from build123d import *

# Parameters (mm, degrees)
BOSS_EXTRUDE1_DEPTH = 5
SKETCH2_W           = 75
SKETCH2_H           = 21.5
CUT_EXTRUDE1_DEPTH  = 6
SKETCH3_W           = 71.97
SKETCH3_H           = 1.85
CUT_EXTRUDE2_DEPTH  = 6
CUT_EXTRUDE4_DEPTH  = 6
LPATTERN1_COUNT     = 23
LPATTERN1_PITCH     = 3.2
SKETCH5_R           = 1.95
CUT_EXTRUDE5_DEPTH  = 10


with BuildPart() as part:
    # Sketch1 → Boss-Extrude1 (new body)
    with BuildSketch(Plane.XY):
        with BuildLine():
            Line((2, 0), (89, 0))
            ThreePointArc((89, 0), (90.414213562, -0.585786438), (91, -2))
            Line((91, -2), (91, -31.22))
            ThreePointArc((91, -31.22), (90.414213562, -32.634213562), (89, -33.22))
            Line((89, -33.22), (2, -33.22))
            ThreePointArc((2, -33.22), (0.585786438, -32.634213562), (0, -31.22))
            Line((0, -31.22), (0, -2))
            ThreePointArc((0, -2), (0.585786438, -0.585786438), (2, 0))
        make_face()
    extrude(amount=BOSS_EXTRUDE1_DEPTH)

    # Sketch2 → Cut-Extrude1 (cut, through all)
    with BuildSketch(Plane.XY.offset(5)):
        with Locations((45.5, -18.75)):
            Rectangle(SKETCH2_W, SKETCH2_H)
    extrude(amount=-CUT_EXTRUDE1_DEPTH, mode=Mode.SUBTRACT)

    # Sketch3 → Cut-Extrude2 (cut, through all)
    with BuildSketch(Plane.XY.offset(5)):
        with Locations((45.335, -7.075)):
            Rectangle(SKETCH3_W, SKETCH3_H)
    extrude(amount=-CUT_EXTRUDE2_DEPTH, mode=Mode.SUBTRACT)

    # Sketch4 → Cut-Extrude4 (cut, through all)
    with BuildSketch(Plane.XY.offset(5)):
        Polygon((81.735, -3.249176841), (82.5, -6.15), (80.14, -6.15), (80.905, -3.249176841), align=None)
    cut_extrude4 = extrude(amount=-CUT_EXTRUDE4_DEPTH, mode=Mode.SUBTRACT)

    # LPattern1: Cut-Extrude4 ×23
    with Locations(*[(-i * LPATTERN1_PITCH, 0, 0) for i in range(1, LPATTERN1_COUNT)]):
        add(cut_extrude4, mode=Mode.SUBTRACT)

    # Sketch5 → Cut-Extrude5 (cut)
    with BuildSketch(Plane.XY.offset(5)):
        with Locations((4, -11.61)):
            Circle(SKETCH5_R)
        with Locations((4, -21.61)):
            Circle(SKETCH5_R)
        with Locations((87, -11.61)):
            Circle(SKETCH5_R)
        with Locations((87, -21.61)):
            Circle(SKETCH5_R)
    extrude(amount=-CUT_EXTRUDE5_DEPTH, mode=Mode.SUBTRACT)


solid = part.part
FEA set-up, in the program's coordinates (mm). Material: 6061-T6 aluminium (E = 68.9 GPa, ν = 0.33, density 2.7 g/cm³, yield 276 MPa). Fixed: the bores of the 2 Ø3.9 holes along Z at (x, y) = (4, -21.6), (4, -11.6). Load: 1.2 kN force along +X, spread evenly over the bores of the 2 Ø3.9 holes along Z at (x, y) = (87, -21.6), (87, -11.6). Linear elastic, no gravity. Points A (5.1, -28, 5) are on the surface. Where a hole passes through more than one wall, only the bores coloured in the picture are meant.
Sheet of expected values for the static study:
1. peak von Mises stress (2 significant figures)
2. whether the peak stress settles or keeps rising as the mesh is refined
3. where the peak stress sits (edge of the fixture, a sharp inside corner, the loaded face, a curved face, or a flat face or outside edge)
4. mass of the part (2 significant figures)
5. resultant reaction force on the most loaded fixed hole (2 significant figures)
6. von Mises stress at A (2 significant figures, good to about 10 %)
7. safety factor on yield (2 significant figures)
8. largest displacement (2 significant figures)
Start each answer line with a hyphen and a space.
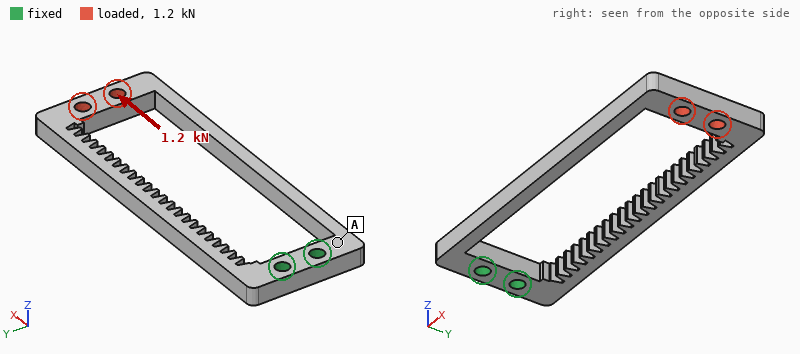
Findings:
- 140 MPa
- settles
- a flat face or outside edge
- 15 g
- 600 N
- 41 MPa
- 1.9
- 0.11 mm
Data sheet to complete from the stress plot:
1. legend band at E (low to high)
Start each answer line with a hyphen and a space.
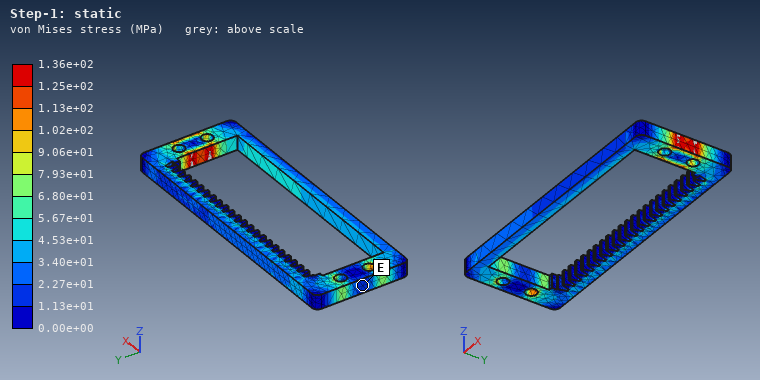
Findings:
- 1.13e+01 to 2.27e+01 MPa
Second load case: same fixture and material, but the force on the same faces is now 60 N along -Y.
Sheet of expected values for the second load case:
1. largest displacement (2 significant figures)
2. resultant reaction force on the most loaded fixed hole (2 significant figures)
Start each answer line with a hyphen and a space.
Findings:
- 0.97 mm
- 170 N
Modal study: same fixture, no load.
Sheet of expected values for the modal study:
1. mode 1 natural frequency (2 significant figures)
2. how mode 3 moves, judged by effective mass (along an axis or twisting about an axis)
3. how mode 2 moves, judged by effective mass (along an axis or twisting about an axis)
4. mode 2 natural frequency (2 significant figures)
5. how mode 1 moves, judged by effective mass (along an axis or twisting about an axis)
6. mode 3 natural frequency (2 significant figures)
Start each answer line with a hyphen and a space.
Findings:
- 360 Hz
- twisting about X
- along Y
- 500 Hz
- along Z
- 1100 Hz
